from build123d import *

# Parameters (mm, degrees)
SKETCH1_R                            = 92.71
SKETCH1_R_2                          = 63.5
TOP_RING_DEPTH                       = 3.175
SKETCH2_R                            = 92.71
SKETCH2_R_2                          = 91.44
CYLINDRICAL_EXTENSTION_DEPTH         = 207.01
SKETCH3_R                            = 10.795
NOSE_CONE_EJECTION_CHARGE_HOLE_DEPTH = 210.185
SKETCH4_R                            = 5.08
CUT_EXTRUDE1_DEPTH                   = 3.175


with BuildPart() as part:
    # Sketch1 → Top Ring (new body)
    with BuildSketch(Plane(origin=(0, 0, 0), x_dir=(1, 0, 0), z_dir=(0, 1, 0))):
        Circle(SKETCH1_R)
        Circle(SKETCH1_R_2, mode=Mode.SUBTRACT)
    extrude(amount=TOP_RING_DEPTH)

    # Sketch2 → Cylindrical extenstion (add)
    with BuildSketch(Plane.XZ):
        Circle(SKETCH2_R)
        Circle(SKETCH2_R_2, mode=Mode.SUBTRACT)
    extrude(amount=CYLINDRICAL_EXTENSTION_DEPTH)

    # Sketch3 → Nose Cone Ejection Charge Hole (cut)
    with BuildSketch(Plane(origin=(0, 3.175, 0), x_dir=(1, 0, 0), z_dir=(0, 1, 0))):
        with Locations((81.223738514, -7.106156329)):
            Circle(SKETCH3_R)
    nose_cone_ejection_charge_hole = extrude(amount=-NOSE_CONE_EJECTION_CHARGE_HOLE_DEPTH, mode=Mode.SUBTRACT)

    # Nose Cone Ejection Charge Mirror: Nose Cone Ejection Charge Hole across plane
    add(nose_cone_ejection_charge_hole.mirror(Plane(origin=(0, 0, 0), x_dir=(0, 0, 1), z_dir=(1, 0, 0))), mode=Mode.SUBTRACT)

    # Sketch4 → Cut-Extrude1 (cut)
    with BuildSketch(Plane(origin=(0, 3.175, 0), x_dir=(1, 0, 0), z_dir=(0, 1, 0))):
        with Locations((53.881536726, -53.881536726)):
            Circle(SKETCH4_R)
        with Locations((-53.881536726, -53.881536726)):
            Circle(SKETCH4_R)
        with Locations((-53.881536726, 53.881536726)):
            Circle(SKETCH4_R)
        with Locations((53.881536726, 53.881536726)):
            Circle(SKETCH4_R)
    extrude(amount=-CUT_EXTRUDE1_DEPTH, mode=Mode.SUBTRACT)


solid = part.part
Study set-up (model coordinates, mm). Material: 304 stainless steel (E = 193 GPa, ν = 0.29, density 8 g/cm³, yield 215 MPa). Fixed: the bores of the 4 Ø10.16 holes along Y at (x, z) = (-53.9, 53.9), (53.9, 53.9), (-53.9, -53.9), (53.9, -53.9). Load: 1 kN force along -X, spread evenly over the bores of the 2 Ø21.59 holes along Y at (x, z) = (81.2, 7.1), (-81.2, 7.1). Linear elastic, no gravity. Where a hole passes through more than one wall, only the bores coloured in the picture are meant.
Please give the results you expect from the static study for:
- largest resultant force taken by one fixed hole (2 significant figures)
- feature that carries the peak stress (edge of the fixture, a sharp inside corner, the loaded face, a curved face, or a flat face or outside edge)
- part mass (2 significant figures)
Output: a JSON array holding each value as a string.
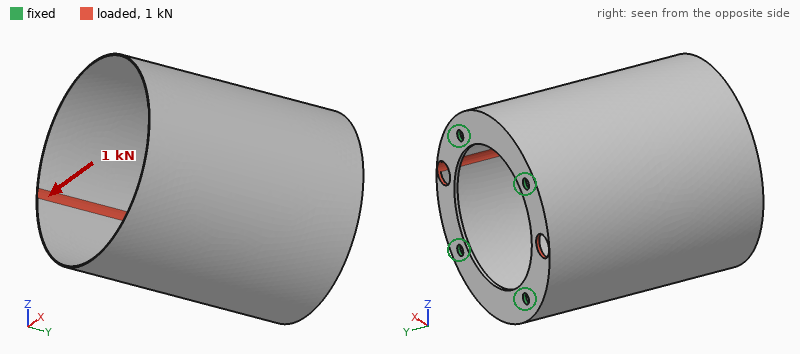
["710 N", "the loaded face", "1.5 kg"]
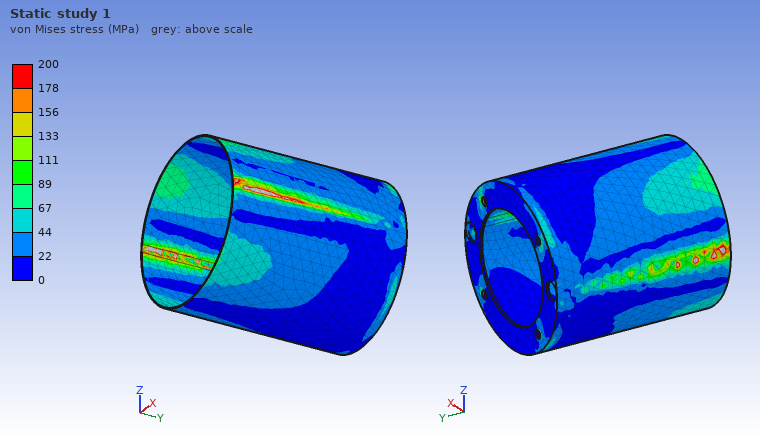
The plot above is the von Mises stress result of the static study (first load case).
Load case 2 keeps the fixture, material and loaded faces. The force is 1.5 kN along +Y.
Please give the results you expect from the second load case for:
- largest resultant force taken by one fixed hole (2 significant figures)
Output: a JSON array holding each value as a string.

["430 N"]
